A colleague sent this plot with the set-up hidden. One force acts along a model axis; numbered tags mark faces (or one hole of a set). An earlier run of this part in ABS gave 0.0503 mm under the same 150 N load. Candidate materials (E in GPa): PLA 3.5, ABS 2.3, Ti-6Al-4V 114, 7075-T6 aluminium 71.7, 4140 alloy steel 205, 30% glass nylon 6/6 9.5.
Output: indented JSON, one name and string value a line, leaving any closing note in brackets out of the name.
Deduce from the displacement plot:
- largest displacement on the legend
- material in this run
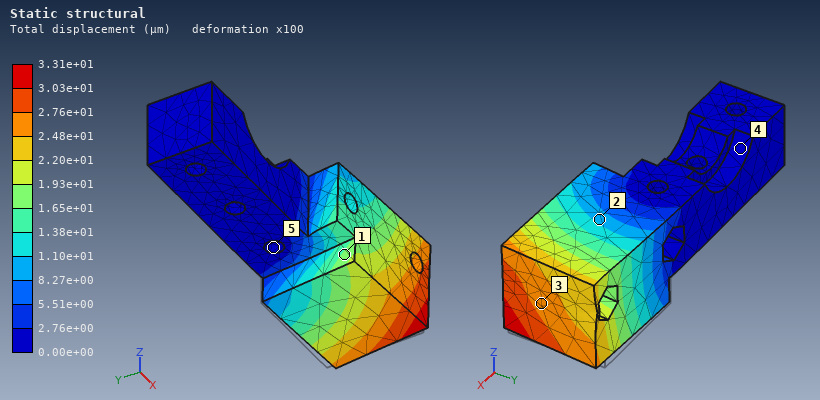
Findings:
{
  "largest displacement on the legend": "3.31e+01 µm",
  "material in this run": "PLA"
}
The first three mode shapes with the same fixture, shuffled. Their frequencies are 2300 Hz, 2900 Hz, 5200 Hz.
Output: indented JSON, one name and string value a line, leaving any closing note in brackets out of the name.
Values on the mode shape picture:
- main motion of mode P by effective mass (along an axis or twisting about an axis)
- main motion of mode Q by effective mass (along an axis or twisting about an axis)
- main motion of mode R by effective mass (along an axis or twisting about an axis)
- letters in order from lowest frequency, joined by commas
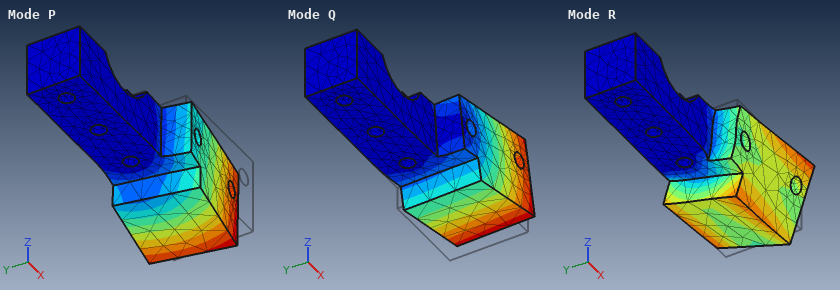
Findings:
{
  "main motion of mode P by effective mass": "along Y",
  "main motion of mode Q by effective mass": "along Z",
  "main motion of mode R by effective mass": "twisting about X",
  "letters in order from lowest frequency, joined by commas": "P, Q, R"
}
